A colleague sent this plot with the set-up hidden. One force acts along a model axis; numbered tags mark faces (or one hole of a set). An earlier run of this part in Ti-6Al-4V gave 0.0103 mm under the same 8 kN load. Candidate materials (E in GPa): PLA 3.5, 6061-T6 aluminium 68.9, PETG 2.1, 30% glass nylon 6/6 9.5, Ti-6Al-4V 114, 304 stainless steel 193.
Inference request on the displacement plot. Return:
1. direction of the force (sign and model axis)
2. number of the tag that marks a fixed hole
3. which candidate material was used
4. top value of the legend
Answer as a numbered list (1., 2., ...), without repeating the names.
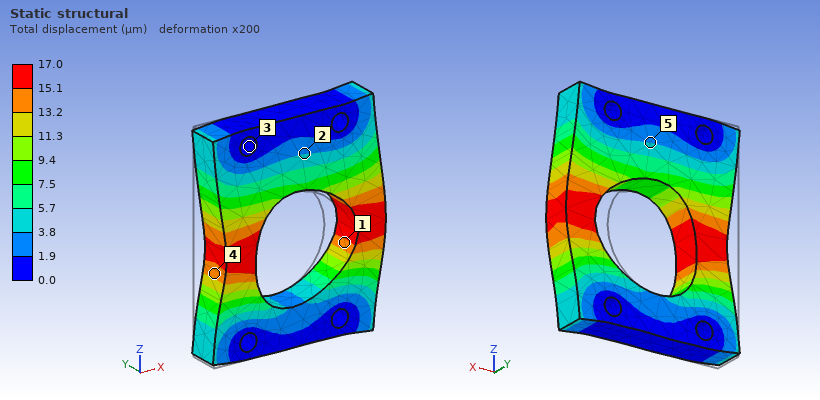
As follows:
1. +X
2. 3
3. 6061-T6 aluminium
4. 17.0 µm
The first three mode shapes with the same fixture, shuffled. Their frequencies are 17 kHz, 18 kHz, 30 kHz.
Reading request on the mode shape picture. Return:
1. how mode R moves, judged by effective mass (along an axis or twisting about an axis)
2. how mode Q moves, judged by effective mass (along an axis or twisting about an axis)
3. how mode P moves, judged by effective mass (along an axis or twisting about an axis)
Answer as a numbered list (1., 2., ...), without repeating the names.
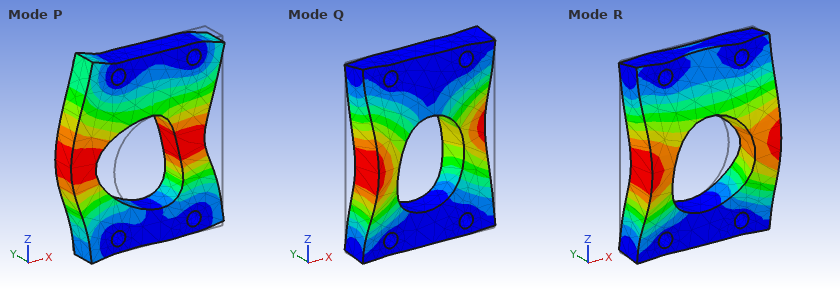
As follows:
1. along Y
2. twisting about Z
3. along X
